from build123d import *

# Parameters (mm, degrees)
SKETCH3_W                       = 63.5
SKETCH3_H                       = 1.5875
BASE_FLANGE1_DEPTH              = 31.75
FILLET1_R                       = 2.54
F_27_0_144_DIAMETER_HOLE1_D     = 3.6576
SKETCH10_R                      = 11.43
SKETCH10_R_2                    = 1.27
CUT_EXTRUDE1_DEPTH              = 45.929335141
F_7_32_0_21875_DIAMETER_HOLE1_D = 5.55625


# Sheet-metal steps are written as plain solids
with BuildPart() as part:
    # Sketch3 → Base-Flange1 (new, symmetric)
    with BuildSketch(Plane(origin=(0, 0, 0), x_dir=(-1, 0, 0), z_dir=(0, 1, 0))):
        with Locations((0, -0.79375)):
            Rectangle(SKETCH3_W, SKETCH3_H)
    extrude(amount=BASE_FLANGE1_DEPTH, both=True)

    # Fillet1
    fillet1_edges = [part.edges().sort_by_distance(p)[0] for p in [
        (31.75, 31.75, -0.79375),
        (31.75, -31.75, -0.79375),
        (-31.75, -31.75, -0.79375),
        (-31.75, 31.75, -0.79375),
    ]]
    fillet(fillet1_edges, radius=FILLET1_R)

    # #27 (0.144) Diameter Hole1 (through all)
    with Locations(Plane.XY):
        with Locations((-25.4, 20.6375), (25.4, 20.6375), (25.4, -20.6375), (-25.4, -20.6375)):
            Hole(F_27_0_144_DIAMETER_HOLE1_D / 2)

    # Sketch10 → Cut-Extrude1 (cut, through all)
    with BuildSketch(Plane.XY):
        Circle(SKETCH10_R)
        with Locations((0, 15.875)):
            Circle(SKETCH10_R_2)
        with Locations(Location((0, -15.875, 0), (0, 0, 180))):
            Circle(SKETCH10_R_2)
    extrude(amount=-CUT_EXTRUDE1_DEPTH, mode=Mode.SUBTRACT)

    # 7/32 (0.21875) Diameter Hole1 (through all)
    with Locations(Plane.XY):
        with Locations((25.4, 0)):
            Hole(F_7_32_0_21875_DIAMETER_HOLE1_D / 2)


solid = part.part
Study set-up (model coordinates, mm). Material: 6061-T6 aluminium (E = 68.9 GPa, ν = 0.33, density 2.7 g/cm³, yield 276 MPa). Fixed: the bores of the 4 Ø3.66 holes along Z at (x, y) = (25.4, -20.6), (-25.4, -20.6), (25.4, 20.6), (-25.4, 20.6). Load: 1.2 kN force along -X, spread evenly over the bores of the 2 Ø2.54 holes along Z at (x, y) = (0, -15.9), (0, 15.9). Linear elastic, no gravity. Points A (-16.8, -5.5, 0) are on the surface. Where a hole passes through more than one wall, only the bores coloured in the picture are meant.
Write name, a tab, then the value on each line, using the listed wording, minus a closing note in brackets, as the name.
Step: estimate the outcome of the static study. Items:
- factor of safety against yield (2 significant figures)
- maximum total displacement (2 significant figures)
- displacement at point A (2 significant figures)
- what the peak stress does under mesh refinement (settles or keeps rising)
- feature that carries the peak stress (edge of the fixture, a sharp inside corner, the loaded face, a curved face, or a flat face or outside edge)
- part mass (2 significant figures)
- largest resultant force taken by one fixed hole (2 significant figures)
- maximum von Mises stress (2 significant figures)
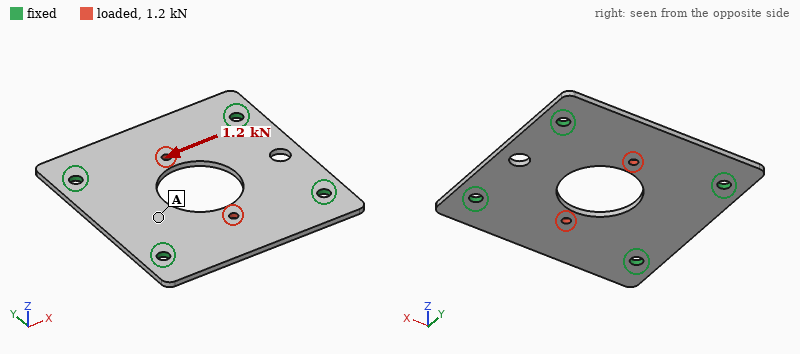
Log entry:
factor of safety against yield	3.4
maximum total displacement	6.6 µm
displacement at point A	2.7 µm
what the peak stress does under mesh refinement	settles
feature that carries the peak stress	the loaded face
part mass	15 g
largest resultant force taken by one fixed hole	310 N
maximum von Mises stress	82 MPa
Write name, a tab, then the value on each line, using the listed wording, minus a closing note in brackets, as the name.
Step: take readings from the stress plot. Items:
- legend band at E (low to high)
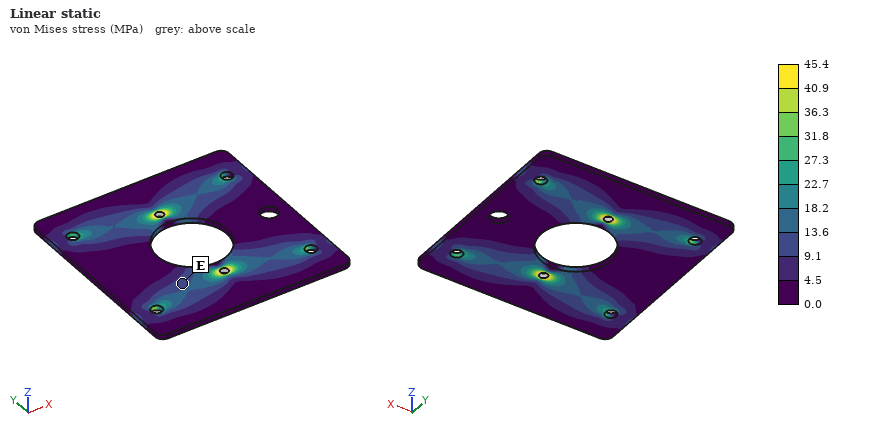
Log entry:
legend band at E	9.1 to 13.6 MPa
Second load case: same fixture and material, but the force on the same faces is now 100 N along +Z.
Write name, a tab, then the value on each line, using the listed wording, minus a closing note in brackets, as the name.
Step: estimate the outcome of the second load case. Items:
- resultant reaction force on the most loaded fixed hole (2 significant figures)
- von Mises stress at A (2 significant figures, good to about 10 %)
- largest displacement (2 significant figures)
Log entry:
resultant reaction force on the most loaded fixed hole	25 N
von Mises stress at A	9.3 MPa
largest displacement	93 µm
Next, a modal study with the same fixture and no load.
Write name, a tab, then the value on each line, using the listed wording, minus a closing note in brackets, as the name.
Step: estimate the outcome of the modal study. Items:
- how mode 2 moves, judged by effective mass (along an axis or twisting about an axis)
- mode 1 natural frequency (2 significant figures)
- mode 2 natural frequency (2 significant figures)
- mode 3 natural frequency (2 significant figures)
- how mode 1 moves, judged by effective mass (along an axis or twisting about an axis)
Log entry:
how mode 2 moves, judged by effective mass	twisting about X
mode 1 natural frequency	3000 Hz
mode 2 natural frequency	3400 Hz
mode 3 natural frequency	4000 Hz
how mode 1 moves, judged by effective mass	along Z
